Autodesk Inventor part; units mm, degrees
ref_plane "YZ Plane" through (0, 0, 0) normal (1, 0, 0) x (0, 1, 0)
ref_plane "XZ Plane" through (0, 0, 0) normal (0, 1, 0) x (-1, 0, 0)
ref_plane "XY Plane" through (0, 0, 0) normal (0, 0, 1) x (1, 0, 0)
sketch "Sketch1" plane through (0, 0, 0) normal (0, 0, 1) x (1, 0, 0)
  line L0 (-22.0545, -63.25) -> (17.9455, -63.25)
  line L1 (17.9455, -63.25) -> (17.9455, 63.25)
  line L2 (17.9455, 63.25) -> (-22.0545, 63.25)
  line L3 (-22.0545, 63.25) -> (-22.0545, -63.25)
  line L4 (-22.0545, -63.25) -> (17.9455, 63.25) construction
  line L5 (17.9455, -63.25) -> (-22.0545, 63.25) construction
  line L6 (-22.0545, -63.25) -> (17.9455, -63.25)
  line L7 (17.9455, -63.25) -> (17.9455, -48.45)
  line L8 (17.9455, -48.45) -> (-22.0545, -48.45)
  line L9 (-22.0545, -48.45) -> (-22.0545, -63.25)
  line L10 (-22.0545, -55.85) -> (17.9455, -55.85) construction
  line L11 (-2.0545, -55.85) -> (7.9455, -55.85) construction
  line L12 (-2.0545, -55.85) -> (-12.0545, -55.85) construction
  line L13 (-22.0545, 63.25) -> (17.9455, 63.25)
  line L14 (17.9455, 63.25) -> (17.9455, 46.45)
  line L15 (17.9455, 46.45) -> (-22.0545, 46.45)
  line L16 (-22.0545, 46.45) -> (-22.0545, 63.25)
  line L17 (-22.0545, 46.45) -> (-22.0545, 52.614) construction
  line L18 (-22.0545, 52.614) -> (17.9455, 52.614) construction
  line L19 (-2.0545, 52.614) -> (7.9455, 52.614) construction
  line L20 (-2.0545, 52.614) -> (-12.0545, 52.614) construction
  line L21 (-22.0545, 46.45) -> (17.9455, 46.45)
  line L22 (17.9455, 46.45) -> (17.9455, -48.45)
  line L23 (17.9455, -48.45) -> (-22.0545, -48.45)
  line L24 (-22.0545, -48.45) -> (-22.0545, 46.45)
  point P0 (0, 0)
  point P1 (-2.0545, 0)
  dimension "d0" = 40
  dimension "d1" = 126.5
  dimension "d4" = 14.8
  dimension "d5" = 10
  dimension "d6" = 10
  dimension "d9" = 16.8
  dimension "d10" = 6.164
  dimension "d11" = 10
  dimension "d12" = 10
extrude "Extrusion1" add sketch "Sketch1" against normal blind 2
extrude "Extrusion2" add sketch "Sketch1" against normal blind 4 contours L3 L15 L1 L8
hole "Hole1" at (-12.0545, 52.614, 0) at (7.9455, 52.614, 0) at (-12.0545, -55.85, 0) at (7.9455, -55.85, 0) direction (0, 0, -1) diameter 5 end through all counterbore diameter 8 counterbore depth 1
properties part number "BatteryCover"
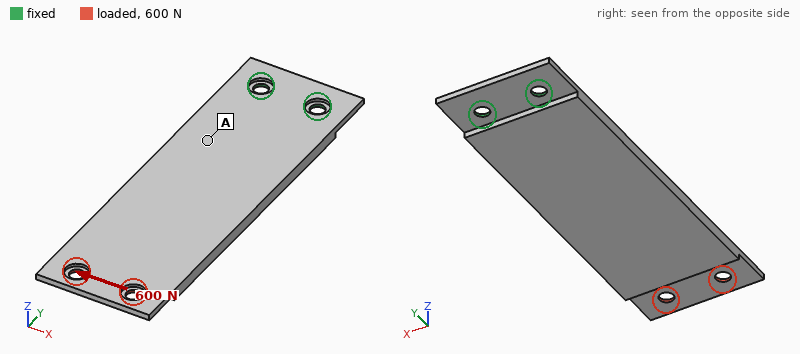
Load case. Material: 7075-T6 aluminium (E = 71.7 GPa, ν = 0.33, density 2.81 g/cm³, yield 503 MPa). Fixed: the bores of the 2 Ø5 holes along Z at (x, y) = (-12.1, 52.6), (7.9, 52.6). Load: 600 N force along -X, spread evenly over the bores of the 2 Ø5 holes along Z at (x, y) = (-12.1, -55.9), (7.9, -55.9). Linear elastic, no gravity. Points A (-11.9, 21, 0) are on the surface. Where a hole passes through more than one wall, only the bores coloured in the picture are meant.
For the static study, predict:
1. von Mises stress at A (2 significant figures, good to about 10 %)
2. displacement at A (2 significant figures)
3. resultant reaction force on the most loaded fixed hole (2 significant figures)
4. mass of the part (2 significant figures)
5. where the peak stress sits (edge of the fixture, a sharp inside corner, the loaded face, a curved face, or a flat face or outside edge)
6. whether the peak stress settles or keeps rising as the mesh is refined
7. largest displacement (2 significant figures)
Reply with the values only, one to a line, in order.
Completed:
27 MPa
0.078 mm
2.9 kN
49 g
edge of the fixture
keeps rising
0.38 mm
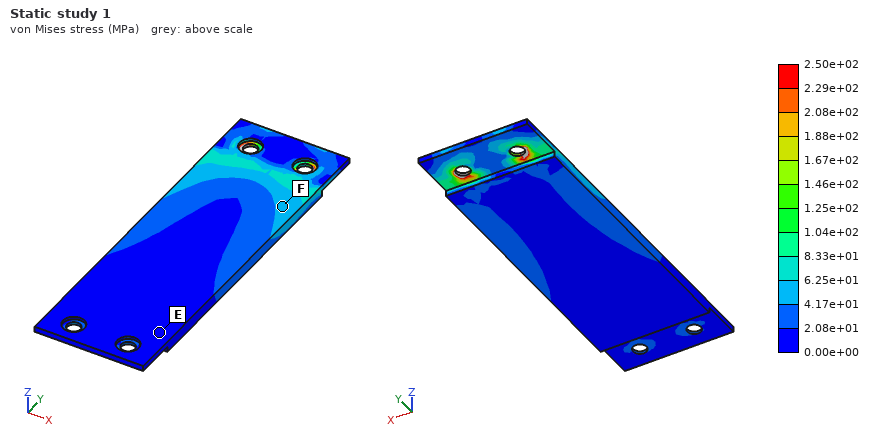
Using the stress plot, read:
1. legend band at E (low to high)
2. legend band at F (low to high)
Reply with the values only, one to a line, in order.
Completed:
0.00e+00 to 2.08e+01 MPa
4.17e+01 to 6.25e+01 MPa
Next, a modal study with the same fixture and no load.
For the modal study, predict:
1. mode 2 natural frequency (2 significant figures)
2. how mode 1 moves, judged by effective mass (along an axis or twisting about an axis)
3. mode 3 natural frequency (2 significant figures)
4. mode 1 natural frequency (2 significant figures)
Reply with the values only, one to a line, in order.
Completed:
1300 Hz
along Z
1300 Hz
150 Hz
